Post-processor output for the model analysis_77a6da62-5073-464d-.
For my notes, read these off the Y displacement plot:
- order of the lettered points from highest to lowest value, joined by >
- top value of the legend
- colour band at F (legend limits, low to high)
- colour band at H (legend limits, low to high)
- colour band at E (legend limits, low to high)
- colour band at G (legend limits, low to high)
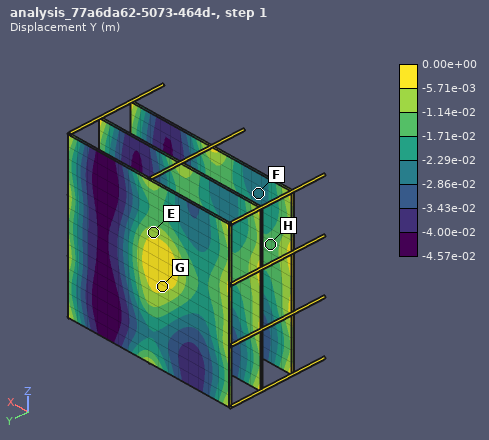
G > E > H > F
0.00e+00 m
-2.86e-02 to -2.29e-02 m
-1.71e-02 to -1.14e-02 m
-1.14e-02 to -5.71e-03 m
-5.71e-03 to 0.00e+00 m
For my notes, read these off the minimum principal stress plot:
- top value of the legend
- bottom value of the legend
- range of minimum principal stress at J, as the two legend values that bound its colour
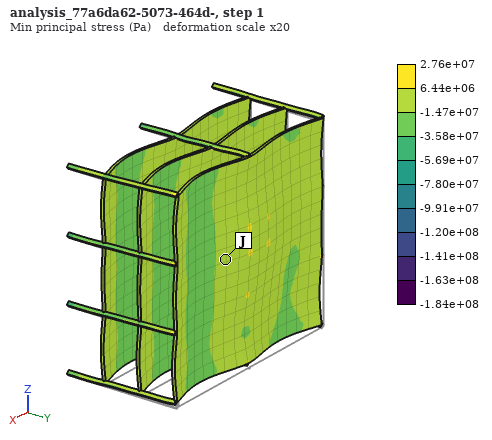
2.76e+07 Pa
-1.84e+08 Pa
-1.47e+07 to 6.44e+06 Pa
